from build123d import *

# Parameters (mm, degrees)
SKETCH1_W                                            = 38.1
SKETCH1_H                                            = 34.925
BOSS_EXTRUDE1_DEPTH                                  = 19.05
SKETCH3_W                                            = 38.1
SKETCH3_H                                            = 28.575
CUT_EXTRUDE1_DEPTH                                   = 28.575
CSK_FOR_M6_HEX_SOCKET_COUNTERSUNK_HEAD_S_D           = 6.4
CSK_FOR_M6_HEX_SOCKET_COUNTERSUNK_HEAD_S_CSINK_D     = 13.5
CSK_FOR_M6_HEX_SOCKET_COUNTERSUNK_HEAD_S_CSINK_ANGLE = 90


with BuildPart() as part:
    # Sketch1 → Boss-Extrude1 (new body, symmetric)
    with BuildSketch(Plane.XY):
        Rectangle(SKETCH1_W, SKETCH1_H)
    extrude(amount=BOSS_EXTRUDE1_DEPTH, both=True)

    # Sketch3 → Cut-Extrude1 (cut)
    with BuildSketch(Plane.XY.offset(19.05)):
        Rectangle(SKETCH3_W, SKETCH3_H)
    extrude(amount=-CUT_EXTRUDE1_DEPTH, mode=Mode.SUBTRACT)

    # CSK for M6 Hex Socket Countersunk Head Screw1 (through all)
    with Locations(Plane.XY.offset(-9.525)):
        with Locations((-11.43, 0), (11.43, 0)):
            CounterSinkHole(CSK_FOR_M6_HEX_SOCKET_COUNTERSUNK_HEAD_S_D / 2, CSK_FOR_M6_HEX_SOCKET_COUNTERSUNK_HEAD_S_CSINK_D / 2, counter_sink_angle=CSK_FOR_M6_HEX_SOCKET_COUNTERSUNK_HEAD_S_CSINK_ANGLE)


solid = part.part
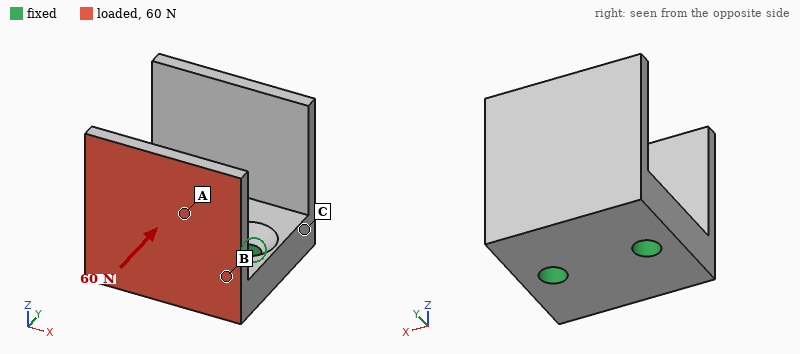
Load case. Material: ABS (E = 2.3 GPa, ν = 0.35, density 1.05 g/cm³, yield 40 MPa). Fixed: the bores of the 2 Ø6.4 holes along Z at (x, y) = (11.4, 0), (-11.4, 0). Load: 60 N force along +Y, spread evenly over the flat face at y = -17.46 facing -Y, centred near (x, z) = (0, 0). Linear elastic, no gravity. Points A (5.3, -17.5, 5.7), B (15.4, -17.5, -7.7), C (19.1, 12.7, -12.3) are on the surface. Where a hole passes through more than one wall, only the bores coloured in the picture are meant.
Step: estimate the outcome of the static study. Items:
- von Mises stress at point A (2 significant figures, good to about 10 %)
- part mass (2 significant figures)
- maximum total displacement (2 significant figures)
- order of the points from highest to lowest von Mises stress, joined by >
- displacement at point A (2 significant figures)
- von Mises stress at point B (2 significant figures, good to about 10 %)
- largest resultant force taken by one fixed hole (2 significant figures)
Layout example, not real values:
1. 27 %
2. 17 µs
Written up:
1. 2.0 MPa
2. 20 g
3. 0.75 mm
4. B > A > C
5. 0.34 mm
6. 7.5 MPa
7. 30 N
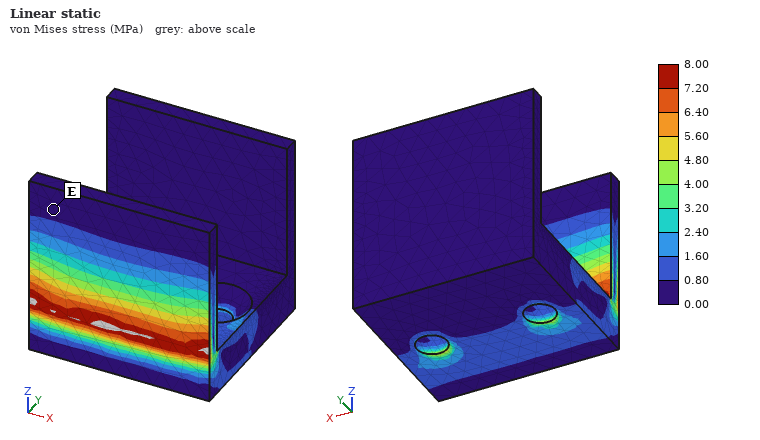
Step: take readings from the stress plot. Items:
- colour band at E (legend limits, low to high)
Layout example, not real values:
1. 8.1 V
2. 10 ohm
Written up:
1. 0.00 to 0.80 MPa
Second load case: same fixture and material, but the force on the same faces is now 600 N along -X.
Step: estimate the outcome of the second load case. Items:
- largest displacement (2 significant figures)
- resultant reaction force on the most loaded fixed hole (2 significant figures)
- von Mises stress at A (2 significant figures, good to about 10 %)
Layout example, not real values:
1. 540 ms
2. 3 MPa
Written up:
1. 0.60 mm
2. 600 N
3. 7.3 MPa
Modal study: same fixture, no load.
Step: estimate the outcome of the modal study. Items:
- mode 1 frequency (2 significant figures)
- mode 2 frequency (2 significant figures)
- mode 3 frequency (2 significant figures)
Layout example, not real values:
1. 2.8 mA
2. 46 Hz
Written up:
1. 790 Hz
2. 820 Hz
3. 1600 Hz
